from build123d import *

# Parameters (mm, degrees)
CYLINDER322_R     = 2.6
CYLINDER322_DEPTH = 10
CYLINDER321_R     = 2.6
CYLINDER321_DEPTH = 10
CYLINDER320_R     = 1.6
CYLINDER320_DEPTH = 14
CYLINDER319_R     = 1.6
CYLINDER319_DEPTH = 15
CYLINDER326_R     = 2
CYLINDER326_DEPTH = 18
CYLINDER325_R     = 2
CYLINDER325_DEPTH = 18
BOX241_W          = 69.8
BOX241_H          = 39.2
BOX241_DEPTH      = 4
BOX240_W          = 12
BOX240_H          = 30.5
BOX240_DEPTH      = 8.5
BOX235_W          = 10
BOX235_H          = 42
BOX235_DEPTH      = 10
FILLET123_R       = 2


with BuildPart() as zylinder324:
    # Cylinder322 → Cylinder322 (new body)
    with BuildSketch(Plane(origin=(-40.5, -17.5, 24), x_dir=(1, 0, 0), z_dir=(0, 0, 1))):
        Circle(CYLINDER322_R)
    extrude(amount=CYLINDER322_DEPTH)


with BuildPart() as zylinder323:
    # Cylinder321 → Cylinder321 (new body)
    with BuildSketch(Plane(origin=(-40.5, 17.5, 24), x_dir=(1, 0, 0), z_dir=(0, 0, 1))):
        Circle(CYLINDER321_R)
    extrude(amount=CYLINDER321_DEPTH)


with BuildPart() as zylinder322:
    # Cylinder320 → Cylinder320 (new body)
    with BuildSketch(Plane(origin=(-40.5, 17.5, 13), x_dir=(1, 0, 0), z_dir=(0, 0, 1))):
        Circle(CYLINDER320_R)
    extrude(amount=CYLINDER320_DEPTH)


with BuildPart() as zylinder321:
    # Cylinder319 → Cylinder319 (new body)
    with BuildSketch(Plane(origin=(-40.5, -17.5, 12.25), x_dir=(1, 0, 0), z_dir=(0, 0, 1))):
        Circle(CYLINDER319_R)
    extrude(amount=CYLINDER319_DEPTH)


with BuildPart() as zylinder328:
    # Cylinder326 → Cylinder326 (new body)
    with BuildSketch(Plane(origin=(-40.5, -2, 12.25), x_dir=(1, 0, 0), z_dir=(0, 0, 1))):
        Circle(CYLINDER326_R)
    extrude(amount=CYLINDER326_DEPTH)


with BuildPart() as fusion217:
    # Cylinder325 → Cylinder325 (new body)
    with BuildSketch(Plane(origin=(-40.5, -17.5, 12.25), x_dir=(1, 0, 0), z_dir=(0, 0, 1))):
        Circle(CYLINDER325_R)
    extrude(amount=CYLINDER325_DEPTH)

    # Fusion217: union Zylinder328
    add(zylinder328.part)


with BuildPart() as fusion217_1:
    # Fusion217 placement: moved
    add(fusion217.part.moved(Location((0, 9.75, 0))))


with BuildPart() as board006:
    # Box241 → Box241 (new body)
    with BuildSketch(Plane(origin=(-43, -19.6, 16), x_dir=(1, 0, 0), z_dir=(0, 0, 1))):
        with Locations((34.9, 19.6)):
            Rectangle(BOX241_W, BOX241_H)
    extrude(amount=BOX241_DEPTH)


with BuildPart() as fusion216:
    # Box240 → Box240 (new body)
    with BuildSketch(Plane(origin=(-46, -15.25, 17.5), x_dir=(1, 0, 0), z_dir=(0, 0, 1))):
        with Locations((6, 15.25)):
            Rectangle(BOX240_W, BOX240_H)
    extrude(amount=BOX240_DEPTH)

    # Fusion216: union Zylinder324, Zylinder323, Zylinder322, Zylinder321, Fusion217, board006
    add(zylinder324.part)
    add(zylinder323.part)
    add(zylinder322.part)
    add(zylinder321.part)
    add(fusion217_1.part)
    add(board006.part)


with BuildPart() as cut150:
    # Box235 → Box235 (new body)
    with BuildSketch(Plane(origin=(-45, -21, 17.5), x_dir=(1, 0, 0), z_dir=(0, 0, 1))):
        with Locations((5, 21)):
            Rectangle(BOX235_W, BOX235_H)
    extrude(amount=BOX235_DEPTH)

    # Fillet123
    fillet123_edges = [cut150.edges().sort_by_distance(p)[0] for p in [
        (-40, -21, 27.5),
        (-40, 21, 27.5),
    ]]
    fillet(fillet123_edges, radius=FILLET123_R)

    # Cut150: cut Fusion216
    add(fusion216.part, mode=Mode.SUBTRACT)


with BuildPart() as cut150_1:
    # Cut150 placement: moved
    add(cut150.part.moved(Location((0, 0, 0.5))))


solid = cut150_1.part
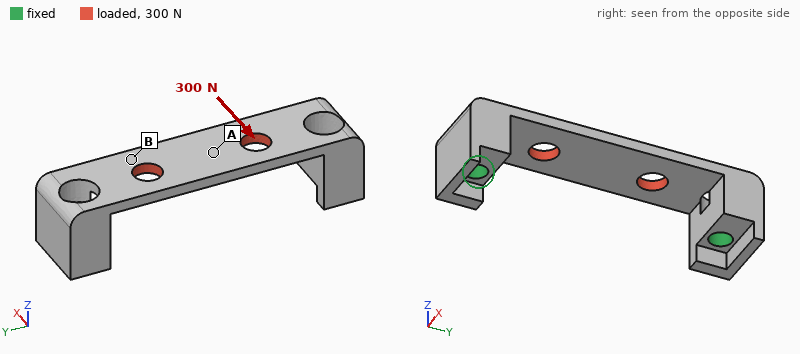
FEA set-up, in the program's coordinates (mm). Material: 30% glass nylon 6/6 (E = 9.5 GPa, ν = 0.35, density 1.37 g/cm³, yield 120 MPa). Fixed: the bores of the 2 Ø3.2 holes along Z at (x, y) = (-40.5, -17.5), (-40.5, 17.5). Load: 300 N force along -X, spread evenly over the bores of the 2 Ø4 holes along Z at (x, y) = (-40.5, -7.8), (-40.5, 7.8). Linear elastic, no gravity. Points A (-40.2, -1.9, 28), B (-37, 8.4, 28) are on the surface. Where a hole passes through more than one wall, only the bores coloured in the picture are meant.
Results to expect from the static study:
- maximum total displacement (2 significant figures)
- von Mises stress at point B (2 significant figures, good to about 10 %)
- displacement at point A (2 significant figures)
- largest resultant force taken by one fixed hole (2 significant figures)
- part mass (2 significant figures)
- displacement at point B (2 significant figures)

0.15 mm
24 MPa
0.15 mm
150 N
1.6 g
0.11 mm
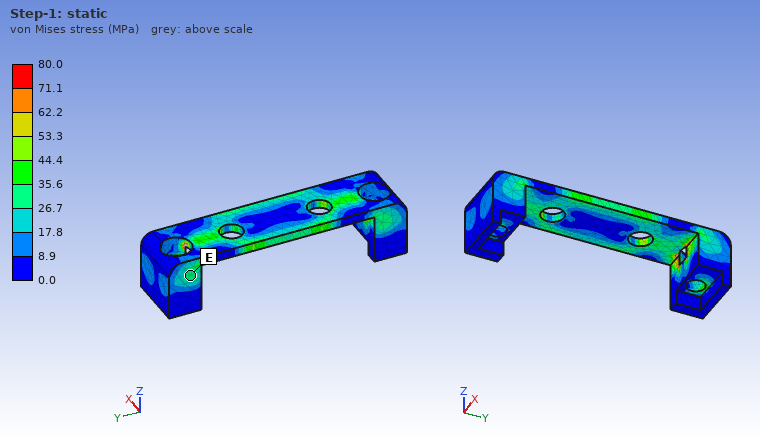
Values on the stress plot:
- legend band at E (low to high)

26.7 to 35.6 MPa
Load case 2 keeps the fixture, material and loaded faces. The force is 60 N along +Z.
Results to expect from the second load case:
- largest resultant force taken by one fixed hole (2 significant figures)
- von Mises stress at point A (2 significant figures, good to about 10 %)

41 N
17 MPa
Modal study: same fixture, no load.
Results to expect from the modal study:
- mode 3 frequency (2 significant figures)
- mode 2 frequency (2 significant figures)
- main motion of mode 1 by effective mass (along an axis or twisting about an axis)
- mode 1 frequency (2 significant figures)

9400 Hz
7600 Hz
along Z
3600 Hz
